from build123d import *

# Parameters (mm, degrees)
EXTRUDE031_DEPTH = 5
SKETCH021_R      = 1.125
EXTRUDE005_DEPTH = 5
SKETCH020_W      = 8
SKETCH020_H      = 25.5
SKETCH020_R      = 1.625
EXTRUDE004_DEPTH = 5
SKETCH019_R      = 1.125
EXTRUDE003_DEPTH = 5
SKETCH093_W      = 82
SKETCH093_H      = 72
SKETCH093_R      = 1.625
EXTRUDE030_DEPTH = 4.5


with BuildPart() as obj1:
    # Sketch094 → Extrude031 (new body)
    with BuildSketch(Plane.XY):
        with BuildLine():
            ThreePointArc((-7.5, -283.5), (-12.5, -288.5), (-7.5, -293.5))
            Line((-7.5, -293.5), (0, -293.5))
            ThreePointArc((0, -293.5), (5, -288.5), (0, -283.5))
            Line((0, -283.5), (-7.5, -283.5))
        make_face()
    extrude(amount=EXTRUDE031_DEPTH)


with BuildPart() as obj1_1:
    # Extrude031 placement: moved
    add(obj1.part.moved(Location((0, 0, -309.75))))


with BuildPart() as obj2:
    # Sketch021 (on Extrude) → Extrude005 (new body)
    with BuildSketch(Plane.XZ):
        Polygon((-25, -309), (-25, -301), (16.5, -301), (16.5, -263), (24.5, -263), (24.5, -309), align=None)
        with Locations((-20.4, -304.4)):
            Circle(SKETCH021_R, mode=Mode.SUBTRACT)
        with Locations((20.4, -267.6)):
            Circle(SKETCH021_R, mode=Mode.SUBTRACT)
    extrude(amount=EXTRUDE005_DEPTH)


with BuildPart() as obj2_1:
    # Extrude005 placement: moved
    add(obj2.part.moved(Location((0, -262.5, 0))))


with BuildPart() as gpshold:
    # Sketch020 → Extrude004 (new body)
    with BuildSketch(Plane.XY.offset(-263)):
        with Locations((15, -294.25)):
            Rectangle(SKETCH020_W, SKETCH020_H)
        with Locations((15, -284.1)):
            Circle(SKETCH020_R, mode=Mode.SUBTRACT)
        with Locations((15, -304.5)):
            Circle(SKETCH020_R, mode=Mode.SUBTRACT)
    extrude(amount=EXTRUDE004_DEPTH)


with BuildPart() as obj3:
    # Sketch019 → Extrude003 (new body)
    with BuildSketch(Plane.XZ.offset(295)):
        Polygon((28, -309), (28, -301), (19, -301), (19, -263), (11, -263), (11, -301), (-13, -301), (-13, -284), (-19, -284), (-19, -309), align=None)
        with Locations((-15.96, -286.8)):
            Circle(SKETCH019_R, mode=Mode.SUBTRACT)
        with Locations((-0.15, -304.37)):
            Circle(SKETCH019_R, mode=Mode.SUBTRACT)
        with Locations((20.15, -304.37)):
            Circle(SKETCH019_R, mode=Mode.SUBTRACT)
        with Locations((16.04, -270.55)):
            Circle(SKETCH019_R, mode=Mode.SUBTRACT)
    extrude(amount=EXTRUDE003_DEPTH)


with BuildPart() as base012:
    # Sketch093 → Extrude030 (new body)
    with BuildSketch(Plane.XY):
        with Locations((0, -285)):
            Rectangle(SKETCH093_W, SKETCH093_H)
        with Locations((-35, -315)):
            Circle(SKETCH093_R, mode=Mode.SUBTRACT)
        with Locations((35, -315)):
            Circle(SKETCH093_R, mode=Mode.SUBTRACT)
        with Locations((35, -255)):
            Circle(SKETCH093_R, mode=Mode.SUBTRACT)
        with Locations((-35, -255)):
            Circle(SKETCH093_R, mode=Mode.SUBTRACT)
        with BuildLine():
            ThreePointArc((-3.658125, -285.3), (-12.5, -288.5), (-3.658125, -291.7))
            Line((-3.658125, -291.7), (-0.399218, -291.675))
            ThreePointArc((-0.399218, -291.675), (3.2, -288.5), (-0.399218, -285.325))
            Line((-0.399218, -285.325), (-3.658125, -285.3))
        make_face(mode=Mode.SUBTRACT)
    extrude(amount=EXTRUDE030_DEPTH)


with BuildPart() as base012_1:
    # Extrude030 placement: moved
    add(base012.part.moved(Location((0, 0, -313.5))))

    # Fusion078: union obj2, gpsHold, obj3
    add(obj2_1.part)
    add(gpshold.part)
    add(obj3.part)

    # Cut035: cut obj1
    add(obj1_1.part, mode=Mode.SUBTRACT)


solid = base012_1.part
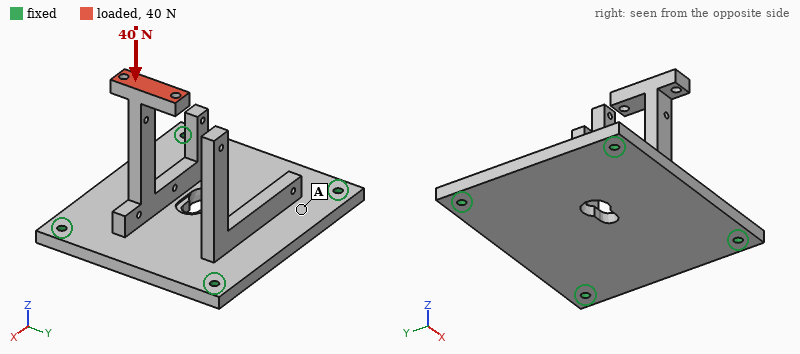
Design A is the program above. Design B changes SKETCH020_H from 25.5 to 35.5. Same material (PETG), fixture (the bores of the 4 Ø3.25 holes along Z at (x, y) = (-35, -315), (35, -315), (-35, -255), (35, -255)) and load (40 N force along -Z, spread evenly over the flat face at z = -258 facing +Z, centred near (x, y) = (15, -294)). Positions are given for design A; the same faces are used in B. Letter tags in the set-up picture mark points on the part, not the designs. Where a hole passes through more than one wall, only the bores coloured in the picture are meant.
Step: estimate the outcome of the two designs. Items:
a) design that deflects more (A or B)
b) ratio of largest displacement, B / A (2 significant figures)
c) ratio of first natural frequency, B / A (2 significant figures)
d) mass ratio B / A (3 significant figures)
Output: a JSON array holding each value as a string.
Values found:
["B", "1.1", "0.86", "1.01"]
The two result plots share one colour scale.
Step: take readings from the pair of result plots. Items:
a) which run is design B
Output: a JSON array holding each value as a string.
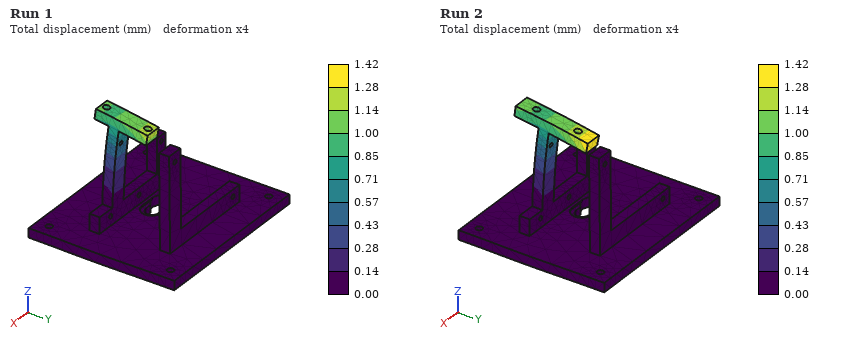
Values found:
["Run 2"]
